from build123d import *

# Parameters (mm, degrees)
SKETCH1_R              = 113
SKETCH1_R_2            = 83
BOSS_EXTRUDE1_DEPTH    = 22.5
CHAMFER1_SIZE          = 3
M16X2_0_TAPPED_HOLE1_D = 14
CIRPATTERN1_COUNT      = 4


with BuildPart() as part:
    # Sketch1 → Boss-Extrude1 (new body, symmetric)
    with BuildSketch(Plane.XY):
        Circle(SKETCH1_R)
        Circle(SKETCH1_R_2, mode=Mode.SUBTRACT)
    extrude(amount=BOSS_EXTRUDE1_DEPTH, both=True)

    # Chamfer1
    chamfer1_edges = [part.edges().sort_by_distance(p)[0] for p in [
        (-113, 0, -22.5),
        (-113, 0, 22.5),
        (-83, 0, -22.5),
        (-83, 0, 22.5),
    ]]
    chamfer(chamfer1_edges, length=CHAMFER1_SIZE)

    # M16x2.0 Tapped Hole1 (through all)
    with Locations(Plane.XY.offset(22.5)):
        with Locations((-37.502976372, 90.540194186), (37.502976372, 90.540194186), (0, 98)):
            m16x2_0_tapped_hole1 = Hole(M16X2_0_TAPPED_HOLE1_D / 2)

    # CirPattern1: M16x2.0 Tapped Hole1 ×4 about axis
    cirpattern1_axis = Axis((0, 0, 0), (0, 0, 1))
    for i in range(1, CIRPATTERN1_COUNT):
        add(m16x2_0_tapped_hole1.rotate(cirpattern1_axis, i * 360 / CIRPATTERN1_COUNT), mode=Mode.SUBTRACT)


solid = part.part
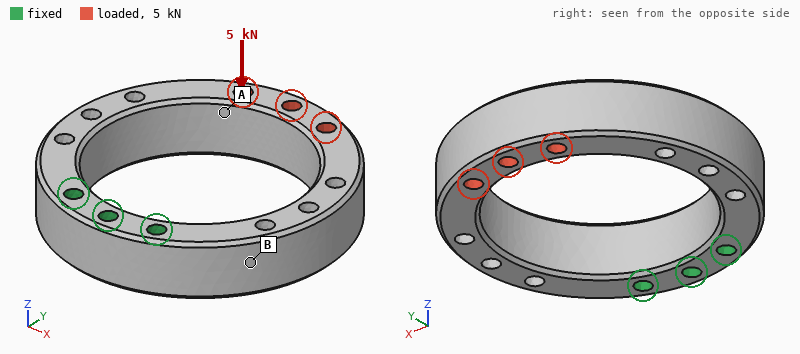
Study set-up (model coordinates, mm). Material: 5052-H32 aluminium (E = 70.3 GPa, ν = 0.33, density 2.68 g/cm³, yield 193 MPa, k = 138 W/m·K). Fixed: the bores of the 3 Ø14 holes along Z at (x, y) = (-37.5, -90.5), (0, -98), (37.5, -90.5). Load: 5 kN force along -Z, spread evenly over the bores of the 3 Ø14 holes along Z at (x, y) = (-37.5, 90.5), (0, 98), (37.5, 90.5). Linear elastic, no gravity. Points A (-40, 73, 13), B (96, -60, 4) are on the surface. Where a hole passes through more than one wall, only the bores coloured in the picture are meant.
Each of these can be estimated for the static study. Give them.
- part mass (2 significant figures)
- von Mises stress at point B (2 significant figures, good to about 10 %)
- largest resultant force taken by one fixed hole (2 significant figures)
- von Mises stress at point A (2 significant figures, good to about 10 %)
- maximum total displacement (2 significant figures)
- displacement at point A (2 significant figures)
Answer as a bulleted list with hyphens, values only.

- 2.0 kg
- 29 MPa
- 2.7 kN
- 9.5 MPa
- 0.91 mm
- 0.66 mm
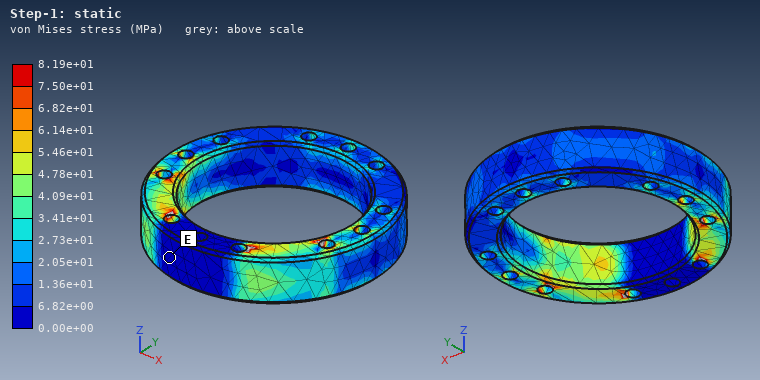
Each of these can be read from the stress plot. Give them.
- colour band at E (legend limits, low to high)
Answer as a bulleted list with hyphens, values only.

- 0.00e+00 to 6.82e+00 MPa
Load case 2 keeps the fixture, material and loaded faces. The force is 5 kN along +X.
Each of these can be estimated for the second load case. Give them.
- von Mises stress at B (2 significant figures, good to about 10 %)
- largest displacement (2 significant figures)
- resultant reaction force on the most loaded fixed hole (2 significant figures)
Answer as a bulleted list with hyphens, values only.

- 21 MPa
- 0.40 mm
- 5.6 kN
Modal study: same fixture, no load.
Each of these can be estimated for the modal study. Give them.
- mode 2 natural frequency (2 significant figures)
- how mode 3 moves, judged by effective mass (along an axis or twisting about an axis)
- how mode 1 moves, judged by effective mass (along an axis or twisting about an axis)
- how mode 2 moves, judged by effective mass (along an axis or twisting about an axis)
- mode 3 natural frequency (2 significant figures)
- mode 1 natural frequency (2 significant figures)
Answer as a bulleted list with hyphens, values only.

- 610 Hz
- twisting about Y
- along Z
- along X
- 1300 Hz
- 500 Hz
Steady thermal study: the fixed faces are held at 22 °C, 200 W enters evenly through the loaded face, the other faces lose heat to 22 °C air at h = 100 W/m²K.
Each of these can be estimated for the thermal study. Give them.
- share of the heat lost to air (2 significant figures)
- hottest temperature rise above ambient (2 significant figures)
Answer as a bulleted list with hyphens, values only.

- 85 %
- 52 K
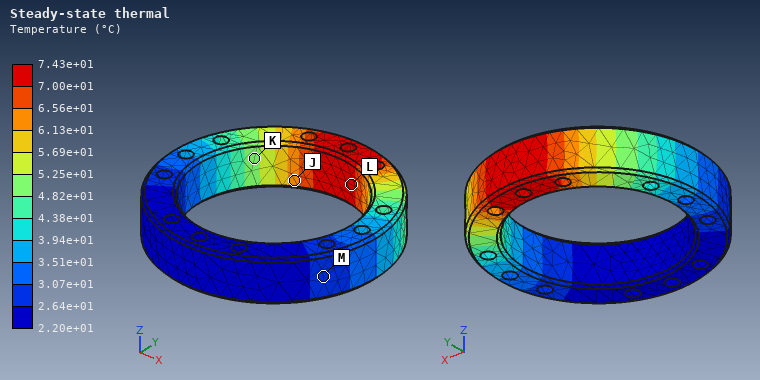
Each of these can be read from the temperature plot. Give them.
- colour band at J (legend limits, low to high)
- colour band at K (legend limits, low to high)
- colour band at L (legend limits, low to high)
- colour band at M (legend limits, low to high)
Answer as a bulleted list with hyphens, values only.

- 6.13e+01 to 6.56e+01 °C
- 4.82e+01 to 5.25e+01 °C
- 7.00e+01 to 7.43e+01 °C
- 2.64e+01 to 3.07e+01 °C
